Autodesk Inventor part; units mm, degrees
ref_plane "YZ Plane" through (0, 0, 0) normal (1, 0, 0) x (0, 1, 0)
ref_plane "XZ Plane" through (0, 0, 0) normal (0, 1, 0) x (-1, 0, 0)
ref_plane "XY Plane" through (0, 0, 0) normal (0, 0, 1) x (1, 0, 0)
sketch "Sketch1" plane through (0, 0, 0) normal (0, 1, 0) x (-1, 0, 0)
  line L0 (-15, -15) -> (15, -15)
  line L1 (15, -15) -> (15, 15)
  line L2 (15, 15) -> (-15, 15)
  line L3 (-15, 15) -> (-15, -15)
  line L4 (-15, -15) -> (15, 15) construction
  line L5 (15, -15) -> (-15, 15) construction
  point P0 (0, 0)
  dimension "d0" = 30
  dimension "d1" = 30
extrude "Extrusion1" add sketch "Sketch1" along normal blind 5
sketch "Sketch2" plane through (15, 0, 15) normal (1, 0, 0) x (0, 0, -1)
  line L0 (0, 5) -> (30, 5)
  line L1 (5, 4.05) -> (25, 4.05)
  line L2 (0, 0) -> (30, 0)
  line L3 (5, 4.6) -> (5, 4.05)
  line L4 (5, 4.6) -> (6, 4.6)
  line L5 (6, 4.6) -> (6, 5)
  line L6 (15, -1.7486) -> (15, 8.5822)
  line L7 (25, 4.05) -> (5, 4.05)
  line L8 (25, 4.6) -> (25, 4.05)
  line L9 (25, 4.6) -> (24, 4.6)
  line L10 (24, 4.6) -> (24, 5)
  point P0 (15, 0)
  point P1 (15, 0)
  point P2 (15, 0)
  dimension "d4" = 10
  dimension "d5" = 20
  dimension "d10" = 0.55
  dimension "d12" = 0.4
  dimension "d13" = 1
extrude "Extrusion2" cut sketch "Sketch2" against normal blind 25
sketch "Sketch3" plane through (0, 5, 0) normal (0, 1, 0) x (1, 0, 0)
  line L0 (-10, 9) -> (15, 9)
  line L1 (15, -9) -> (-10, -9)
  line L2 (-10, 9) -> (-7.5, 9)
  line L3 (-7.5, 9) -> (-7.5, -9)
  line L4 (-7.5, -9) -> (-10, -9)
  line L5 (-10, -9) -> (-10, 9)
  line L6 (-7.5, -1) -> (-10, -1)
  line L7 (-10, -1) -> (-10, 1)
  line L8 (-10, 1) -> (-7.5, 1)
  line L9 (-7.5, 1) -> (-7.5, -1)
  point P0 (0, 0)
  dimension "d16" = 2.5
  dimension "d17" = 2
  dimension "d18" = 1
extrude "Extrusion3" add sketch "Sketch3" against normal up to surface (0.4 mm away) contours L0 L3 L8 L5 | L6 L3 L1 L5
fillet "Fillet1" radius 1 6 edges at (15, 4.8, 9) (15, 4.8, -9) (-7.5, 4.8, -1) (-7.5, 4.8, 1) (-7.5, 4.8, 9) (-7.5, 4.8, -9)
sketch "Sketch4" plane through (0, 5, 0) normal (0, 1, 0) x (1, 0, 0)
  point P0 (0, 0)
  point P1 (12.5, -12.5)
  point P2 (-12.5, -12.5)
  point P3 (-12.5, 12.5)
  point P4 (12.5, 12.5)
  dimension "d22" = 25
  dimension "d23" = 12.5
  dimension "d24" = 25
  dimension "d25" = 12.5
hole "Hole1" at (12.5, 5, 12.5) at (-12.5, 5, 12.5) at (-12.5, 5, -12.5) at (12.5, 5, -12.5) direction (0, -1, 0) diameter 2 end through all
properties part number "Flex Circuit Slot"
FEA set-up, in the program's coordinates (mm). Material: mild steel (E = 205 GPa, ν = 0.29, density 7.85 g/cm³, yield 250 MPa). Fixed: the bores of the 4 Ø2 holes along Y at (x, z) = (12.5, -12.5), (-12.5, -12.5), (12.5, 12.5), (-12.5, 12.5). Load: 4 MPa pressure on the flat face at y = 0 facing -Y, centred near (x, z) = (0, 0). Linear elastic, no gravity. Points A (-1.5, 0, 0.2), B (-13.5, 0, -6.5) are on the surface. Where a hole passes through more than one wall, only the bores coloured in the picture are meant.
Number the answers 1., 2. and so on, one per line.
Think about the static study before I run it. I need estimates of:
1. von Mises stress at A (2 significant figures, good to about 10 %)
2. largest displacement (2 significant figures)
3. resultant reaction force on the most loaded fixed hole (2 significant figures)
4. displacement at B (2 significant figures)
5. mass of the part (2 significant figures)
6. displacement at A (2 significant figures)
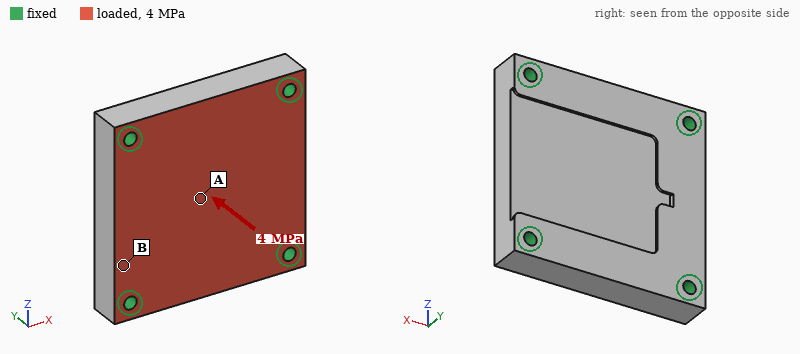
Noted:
1. 42 MPa
2. 9.3 µm
3. 900 N
4. 2.9 µm
5. 31 g
6. 9.2 µm
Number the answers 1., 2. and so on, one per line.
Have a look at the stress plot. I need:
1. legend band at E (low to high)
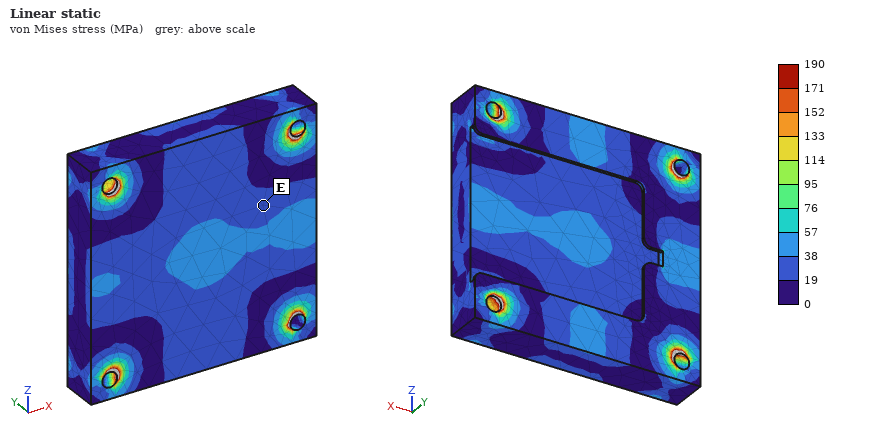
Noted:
1. 19 to 38 MPa
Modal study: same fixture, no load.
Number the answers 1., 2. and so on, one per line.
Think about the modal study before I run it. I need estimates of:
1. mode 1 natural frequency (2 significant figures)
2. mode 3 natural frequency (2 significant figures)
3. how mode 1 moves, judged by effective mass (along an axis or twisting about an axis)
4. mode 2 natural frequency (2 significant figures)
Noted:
1. 22 kHz
2. 35 kHz
3. along Y
4. 35 kHz
